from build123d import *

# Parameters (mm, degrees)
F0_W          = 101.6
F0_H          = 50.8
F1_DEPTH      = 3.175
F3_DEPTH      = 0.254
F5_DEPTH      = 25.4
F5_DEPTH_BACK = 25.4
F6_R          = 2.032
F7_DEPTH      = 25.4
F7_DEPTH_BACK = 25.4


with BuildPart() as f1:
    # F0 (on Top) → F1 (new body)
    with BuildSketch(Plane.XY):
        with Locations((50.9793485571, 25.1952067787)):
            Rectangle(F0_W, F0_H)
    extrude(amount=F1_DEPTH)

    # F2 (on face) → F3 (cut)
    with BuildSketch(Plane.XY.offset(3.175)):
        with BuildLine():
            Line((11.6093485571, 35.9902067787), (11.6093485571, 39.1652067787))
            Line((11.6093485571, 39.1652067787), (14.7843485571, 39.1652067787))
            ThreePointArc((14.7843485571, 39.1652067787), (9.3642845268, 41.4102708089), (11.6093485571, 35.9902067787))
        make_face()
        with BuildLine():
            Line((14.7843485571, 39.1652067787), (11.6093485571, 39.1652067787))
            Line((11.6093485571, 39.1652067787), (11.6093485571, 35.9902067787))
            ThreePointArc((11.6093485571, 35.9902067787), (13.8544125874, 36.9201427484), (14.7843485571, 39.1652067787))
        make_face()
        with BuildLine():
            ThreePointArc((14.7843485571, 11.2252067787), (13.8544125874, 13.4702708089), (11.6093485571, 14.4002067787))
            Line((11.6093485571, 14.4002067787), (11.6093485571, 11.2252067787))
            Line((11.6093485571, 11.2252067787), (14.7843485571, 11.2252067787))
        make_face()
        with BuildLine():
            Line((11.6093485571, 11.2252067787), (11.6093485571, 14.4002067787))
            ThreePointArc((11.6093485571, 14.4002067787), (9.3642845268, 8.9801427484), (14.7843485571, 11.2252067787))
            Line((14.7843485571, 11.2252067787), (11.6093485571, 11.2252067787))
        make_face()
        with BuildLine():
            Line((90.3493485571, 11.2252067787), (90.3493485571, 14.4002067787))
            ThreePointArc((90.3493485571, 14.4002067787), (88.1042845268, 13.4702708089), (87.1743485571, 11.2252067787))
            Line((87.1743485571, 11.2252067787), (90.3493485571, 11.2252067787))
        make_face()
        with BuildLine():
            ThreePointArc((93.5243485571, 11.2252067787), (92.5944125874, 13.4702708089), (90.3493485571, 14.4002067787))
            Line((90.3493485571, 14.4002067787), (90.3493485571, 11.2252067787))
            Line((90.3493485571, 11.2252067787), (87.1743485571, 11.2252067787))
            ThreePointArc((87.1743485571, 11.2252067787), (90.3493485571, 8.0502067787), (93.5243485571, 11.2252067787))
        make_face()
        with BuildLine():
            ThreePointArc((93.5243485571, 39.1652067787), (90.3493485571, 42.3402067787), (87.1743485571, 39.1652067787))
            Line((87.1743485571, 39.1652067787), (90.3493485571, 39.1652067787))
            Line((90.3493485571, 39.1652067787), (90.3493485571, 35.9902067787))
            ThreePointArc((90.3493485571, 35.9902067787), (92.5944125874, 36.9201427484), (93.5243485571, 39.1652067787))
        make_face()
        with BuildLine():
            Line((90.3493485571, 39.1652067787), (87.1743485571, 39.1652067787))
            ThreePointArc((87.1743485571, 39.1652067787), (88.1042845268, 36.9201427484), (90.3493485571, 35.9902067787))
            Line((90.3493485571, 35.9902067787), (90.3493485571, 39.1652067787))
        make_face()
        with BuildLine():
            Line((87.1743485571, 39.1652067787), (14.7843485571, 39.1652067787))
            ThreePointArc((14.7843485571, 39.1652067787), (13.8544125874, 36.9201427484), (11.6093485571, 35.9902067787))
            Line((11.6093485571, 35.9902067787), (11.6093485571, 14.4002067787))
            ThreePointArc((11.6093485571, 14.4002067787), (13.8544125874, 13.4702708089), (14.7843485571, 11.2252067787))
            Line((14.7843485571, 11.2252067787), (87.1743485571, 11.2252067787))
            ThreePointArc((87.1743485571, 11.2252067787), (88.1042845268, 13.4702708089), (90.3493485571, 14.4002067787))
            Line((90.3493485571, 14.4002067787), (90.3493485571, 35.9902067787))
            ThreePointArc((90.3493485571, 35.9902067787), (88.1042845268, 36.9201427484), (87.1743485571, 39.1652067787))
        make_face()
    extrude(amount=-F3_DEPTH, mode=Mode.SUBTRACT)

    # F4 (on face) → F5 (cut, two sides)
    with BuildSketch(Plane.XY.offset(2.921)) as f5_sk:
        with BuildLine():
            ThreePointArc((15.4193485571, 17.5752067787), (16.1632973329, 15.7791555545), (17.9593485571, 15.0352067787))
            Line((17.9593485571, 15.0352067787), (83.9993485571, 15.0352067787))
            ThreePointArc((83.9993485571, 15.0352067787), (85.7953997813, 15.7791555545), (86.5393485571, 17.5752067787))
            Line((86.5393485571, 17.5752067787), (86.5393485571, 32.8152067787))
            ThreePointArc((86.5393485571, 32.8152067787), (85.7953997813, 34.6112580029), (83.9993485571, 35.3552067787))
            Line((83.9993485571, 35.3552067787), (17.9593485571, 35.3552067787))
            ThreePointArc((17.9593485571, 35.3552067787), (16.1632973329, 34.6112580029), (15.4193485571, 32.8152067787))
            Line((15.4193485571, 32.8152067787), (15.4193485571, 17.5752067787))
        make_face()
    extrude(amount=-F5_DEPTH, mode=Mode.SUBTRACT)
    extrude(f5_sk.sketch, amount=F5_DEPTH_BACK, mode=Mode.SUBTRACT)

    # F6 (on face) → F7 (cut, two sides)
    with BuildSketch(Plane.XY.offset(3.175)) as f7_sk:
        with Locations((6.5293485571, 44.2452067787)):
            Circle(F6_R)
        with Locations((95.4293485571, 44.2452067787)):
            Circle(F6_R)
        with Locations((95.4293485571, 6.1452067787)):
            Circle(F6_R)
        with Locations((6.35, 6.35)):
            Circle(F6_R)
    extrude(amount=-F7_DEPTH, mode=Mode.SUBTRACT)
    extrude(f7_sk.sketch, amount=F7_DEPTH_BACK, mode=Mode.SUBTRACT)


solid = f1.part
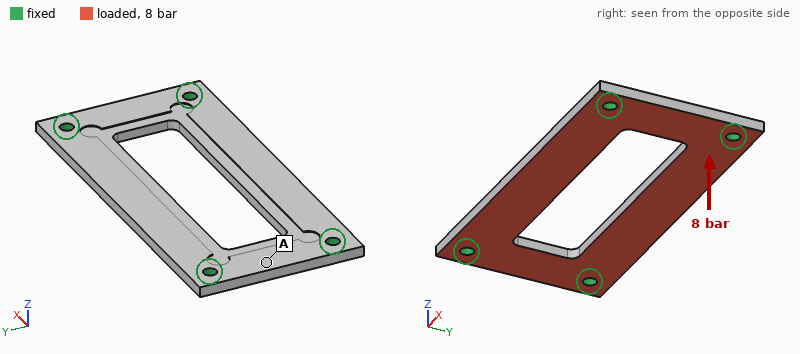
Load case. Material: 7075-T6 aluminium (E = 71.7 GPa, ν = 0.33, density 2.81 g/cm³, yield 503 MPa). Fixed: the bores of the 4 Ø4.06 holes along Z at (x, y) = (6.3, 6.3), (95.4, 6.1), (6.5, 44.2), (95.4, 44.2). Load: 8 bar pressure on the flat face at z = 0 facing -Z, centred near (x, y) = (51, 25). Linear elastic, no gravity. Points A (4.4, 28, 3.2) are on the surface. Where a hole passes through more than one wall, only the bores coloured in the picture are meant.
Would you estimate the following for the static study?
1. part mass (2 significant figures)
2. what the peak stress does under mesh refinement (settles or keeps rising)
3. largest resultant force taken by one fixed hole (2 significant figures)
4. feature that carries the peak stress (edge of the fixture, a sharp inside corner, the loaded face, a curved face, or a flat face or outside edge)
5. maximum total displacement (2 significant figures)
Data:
32 g
keeps rising
740 N
edge of the fixture
0.68 mm
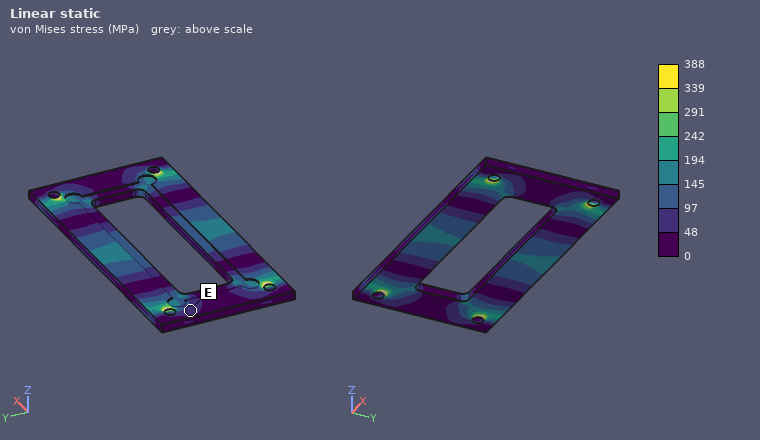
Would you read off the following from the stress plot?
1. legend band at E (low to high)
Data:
48 to 97 MPa
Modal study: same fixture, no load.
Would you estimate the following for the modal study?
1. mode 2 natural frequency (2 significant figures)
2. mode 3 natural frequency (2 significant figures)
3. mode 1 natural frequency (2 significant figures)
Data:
2200 Hz
5800 Hz
2200 Hz
